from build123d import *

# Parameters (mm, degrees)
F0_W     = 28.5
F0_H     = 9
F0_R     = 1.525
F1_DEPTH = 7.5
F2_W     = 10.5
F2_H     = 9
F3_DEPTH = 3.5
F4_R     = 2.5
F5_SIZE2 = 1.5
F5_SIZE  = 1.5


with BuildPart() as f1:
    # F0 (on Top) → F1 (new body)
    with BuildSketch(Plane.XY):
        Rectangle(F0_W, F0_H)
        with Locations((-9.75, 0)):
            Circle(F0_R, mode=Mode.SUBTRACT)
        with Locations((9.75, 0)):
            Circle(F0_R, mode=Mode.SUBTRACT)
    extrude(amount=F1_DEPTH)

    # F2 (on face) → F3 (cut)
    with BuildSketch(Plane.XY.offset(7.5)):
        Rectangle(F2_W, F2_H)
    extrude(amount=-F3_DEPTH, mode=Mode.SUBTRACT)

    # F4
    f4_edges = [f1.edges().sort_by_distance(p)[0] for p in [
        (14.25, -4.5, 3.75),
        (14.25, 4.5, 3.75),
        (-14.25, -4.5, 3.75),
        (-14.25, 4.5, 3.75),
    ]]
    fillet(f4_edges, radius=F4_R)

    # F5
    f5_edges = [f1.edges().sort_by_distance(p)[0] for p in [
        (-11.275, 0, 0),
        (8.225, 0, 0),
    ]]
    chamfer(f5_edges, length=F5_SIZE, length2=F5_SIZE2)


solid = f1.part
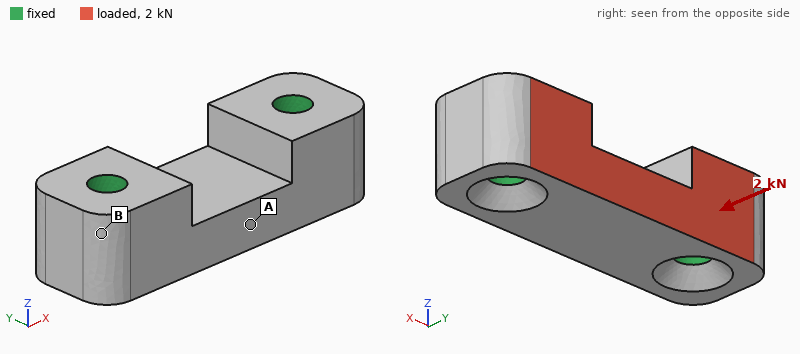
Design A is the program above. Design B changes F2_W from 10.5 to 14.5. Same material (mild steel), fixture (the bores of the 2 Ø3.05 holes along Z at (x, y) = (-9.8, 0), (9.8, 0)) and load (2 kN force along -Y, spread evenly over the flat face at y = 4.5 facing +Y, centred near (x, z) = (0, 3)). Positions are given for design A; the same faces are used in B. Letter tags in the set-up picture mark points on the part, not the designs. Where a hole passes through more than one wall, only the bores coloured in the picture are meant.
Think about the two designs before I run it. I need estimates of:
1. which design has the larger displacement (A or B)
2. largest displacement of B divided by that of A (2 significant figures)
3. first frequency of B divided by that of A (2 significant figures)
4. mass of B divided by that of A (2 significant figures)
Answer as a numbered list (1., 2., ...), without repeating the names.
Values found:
1. B
2. 1.1
3. 0.82
4. 0.91
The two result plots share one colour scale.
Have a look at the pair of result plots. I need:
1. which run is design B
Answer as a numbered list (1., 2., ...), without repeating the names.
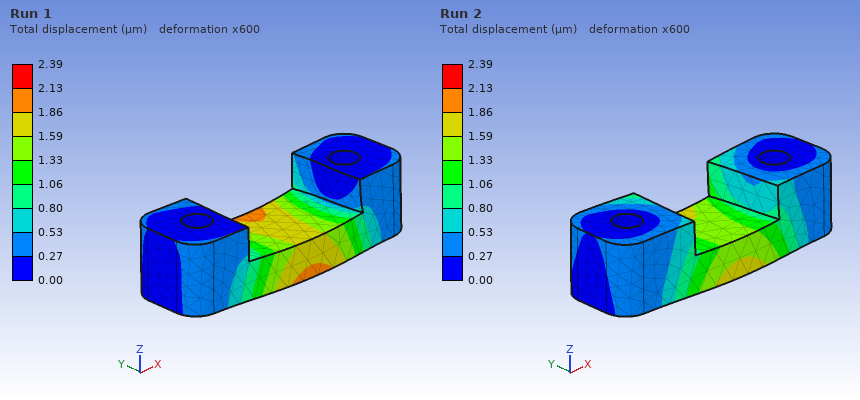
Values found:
1. Run 1
